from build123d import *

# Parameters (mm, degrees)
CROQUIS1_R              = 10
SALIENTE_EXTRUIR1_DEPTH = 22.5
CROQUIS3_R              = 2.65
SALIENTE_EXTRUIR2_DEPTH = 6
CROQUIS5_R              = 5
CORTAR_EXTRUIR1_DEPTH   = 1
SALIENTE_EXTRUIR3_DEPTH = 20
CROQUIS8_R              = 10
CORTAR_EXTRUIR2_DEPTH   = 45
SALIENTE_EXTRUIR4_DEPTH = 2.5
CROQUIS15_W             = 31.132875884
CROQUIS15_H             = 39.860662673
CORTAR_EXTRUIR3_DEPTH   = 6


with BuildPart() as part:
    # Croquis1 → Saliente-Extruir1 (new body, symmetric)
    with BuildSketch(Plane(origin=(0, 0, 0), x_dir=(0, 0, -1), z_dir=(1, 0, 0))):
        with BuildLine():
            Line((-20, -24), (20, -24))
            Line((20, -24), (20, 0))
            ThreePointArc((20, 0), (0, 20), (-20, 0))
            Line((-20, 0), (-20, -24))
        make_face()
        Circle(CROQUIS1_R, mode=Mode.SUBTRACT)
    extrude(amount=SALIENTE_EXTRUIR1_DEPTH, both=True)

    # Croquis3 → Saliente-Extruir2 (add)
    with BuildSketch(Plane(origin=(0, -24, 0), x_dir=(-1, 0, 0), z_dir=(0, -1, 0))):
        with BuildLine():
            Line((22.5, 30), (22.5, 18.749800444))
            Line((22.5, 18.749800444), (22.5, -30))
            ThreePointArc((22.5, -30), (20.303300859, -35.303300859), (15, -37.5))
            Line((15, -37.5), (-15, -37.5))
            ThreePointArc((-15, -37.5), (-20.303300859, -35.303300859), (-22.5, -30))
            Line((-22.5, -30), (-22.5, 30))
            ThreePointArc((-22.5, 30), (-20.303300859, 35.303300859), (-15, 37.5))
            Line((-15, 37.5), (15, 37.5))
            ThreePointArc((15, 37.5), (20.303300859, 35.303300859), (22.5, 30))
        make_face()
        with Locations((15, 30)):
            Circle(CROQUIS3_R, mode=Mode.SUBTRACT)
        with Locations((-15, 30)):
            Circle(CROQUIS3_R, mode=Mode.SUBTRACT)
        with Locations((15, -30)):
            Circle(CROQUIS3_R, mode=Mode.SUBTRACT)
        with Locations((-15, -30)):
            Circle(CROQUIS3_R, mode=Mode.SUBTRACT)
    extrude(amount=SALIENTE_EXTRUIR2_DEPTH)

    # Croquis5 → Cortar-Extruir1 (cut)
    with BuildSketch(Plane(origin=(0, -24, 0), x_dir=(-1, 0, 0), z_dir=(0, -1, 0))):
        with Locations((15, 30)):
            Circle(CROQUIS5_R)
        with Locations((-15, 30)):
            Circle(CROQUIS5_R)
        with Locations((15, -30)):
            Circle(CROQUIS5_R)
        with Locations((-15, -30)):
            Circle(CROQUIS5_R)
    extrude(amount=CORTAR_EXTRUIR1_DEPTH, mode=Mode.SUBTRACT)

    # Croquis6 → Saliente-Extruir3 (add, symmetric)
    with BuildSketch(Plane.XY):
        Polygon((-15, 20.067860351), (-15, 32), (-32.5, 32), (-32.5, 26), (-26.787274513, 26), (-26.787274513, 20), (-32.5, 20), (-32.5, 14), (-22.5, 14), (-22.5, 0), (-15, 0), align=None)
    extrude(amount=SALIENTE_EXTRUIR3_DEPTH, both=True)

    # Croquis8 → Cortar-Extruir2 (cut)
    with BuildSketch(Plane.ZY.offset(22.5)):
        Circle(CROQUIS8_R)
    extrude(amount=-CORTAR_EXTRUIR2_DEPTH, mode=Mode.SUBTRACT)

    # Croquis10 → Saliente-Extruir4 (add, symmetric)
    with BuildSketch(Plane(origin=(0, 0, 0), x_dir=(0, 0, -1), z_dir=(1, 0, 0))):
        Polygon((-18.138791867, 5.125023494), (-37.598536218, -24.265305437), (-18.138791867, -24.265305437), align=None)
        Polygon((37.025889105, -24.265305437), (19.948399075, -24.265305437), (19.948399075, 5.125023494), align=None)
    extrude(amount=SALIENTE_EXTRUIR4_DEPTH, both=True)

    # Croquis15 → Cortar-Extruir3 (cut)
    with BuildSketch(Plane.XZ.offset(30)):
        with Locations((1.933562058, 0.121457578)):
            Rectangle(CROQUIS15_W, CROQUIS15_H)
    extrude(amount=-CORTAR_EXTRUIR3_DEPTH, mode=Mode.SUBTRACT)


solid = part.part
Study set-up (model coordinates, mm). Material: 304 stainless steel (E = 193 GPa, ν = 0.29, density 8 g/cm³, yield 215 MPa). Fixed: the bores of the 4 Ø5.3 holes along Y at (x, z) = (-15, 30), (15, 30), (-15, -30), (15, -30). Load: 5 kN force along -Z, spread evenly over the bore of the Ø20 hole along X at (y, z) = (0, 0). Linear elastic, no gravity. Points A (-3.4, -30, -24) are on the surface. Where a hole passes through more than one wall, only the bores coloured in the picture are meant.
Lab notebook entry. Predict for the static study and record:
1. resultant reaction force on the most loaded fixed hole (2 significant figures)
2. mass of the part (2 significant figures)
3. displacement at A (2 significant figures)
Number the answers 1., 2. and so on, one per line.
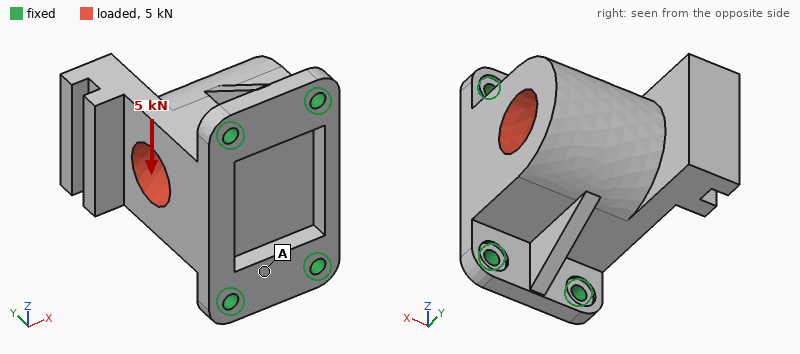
1. 1.9 kN
2. 660 g
3. 3.2 µm
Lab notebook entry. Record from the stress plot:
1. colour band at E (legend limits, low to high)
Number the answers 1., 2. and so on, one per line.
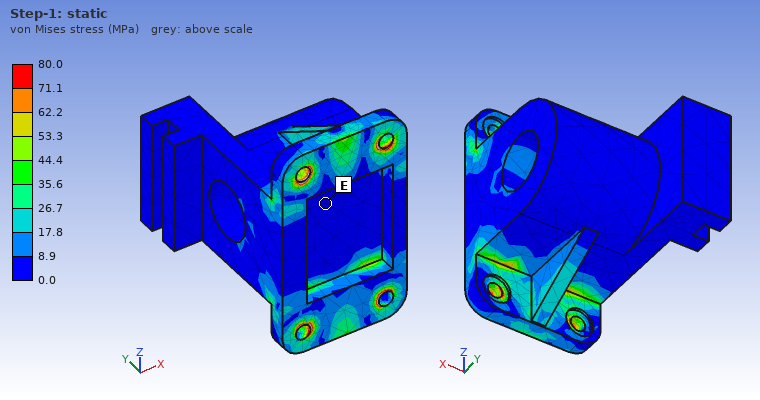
1. 0.0 to 8.9 MPa
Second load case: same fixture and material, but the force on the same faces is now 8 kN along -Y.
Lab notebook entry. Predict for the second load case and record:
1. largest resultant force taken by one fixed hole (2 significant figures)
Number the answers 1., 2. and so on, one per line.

1. 2.5 kN
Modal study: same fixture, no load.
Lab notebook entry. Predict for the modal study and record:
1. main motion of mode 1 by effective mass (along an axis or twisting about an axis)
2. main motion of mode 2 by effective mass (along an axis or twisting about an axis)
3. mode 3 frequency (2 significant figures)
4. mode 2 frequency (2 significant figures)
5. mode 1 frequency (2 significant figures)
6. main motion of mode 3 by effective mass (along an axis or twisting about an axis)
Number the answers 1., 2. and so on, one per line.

1. along X
2. along Z
3. 6100 Hz
4. 4600 Hz
5. 2500 Hz
6. along Y
